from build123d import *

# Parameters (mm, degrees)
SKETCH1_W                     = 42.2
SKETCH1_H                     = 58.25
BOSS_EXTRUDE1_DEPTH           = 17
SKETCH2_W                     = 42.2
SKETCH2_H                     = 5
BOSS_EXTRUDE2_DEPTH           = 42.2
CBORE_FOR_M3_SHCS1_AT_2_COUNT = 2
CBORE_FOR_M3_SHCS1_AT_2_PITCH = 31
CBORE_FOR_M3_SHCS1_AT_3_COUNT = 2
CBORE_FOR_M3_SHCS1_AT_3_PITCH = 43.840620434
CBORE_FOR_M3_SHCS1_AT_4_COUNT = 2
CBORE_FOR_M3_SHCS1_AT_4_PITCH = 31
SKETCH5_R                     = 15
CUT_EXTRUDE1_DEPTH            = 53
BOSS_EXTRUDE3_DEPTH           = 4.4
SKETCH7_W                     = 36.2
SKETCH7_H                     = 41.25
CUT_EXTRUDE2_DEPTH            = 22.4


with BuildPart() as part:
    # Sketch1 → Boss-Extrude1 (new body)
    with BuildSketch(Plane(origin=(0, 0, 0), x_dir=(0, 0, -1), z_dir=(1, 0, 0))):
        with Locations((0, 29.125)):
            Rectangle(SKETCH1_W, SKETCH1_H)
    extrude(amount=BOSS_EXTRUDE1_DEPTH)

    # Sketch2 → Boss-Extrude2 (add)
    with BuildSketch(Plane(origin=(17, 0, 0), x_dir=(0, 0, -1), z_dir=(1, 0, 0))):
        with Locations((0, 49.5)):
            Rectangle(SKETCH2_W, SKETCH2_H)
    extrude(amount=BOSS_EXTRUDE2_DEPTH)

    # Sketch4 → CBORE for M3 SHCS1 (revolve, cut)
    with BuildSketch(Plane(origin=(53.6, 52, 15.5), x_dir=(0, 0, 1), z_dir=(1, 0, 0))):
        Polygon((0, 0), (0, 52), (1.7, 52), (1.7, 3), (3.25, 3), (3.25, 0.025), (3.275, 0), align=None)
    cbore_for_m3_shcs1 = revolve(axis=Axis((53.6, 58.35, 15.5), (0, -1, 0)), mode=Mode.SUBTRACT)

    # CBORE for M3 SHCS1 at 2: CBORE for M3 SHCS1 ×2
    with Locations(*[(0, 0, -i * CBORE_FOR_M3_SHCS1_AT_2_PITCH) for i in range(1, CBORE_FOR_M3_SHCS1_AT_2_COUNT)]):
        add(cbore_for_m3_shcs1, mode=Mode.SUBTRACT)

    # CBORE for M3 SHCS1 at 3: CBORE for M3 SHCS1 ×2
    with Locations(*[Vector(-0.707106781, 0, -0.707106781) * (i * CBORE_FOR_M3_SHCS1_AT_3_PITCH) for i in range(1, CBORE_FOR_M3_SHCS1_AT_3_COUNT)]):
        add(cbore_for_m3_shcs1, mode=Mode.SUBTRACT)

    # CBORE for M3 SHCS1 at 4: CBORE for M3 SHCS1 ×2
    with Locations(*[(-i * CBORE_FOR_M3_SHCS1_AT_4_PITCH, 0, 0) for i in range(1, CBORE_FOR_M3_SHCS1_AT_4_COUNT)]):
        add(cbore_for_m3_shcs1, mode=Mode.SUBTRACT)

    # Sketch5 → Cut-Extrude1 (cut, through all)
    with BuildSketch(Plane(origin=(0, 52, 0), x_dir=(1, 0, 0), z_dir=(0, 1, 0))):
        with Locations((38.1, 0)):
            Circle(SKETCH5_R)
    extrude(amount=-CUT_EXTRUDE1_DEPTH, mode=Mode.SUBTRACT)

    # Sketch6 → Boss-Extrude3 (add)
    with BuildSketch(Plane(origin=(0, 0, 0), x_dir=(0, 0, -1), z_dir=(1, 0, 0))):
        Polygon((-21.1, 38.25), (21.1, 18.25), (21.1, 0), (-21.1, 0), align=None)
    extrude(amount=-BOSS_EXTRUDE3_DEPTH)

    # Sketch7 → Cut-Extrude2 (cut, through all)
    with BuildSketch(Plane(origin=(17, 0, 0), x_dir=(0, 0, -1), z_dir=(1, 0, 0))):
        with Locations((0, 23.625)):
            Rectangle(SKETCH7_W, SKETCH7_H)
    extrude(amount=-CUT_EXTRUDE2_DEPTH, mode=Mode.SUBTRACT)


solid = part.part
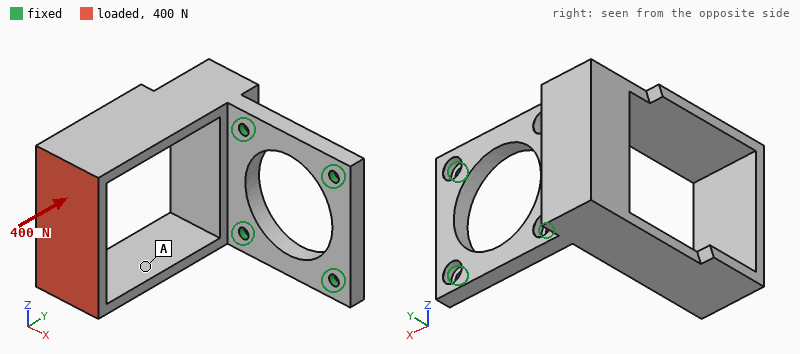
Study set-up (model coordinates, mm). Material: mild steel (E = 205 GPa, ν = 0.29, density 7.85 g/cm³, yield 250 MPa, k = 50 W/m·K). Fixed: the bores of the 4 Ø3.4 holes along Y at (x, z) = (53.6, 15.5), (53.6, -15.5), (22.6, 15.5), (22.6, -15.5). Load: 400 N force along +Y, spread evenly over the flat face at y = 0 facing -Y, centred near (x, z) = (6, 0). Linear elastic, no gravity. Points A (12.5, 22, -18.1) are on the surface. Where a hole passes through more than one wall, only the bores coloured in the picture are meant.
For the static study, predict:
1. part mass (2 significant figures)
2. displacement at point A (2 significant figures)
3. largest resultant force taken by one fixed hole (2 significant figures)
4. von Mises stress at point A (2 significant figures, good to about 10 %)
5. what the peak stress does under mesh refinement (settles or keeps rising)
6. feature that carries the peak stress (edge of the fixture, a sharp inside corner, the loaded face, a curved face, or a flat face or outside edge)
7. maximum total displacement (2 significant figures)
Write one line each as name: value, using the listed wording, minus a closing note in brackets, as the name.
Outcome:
part mass: 180 g
displacement at point A: 36 µm
largest resultant force taken by one fixed hole: 310 N
von Mises stress at point A: 12 MPa
what the peak stress does under mesh refinement: keeps rising
feature that carries the peak stress: edge of the fixture
maximum total displacement: 79 µm
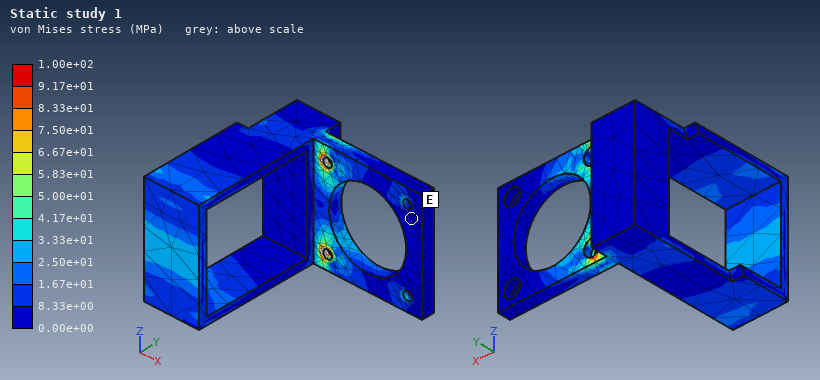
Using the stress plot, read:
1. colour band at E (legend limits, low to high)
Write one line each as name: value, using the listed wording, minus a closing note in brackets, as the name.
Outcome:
colour band at E: 0.00e+00 to 8.33e+00 MPa
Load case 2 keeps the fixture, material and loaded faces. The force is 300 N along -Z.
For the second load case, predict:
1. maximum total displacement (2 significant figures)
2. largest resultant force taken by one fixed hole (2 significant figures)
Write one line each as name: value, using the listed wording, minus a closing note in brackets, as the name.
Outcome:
maximum total displacement: 0.17 mm
largest resultant force taken by one fixed hole: 490 N
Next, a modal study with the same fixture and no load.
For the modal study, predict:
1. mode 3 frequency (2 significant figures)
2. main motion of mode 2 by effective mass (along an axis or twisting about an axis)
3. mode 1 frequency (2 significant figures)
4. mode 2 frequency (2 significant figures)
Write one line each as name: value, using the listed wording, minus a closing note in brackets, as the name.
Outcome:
mode 3 frequency: 3700 Hz
main motion of mode 2 by effective mass: along Z
mode 1 frequency: 1000 Hz
mode 2 frequency: 1100 Hz
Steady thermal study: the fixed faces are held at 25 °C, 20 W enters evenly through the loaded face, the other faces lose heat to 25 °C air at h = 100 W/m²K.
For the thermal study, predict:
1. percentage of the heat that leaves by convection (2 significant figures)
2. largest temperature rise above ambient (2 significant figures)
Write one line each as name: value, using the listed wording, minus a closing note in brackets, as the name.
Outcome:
percentage of the heat that leaves by convection: 89 %
largest temperature rise above ambient: 70 K
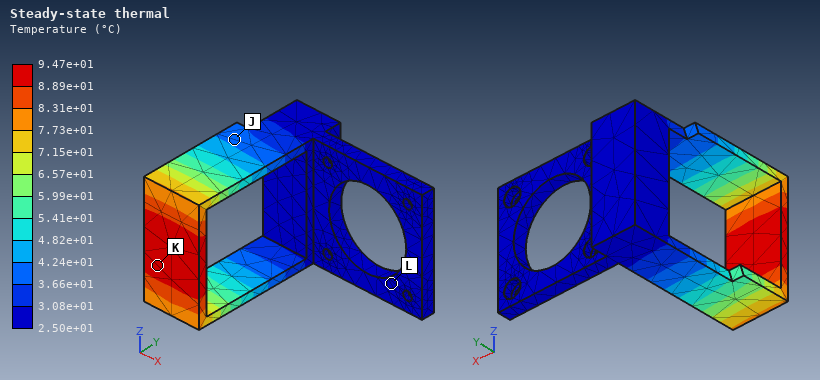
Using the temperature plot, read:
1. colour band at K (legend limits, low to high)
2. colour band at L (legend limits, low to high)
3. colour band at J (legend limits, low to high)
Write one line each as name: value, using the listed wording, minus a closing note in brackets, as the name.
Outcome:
colour band at K: 8.89e+01 to 9.47e+01 °C
colour band at L: 2.50e+01 to 3.08e+01 °C
colour band at J: 3.66e+01 to 4.24e+01 °C
